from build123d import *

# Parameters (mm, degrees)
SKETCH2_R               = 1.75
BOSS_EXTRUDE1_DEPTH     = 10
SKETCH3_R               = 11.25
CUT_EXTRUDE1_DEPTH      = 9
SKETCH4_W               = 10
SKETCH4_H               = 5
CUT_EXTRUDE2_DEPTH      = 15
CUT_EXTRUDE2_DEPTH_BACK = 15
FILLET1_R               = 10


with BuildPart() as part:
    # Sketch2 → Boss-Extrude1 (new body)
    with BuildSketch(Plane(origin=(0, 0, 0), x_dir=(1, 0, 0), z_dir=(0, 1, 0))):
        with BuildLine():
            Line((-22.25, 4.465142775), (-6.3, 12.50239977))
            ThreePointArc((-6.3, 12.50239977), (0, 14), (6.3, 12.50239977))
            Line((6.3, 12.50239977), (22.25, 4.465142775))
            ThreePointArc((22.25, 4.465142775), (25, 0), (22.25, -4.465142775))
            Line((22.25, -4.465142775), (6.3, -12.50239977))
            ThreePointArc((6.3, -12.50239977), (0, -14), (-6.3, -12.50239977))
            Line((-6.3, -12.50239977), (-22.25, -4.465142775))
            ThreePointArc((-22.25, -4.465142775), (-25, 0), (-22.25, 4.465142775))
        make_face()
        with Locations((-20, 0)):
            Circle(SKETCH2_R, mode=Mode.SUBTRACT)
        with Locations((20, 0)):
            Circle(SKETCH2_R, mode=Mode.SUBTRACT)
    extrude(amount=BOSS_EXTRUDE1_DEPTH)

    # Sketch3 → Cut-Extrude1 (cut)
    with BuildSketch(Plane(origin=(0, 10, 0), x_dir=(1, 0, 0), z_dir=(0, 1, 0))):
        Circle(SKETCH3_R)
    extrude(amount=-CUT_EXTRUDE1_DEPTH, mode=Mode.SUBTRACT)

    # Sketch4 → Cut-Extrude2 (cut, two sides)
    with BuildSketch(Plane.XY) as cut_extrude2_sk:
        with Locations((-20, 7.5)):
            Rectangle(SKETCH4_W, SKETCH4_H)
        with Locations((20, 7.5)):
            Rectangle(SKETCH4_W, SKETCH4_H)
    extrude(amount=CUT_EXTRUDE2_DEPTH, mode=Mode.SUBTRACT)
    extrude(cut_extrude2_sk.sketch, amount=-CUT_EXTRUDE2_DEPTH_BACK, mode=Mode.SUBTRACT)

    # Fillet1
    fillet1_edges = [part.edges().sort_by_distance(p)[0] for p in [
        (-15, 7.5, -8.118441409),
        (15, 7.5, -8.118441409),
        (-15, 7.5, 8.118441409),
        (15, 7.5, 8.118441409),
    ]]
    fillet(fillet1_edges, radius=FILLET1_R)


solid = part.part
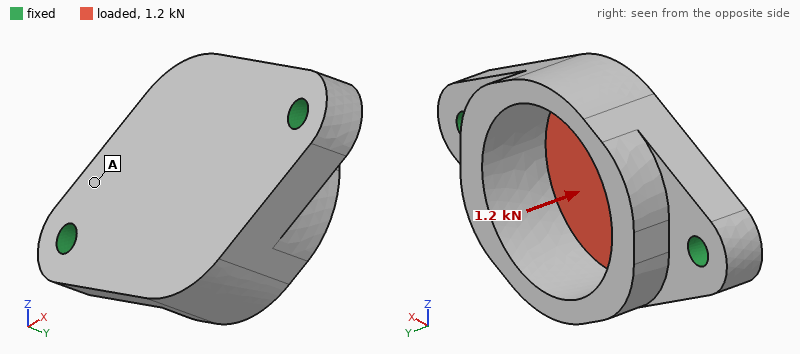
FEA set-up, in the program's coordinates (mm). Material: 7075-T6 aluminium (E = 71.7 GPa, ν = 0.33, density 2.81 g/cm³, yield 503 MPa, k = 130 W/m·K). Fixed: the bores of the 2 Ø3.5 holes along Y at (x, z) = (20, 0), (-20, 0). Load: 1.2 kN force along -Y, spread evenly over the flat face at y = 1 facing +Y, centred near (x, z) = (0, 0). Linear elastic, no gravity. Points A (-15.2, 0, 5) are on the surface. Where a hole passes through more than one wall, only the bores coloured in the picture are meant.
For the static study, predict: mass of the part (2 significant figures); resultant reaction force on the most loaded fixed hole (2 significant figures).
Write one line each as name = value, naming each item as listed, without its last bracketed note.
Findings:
mass of the part = 12 g
resultant reaction force on the most loaded fixed hole = 610 N
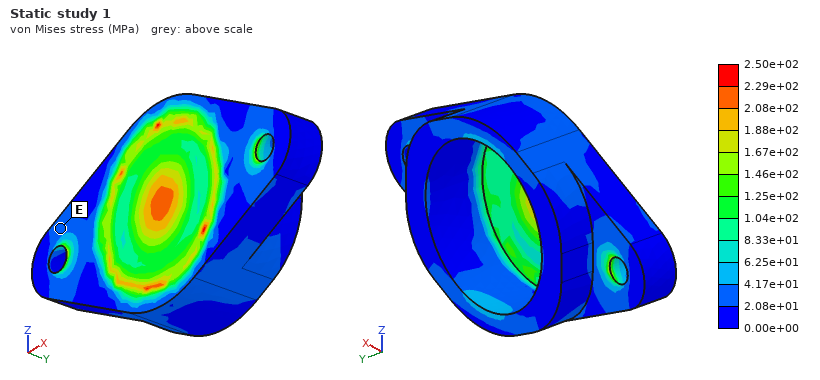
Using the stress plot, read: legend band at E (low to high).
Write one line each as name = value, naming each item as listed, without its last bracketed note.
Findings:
legend band at E = 2.08e+01 to 4.17e+01 MPa
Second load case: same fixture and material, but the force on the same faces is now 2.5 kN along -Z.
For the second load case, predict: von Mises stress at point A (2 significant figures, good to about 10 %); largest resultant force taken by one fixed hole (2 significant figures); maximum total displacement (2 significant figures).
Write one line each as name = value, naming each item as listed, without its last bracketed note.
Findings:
von Mises stress at point A = 42 MPa
largest resultant force taken by one fixed hole = 1.3 kN
maximum total displacement = 28 µm
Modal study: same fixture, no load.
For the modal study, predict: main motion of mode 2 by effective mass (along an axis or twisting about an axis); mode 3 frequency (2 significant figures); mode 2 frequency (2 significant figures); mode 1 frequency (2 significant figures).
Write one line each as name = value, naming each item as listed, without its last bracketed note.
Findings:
main motion of mode 2 by effective mass = along Y
mode 3 frequency = 19 kHz
mode 2 frequency = 13 kHz
mode 1 frequency = 11 kHz
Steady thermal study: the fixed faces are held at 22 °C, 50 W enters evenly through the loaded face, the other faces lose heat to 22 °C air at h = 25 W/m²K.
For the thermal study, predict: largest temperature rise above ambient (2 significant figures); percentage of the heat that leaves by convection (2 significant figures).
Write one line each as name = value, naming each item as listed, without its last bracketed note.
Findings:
largest temperature rise above ambient = 63 K
percentage of the heat that leaves by convection = 3.7 %
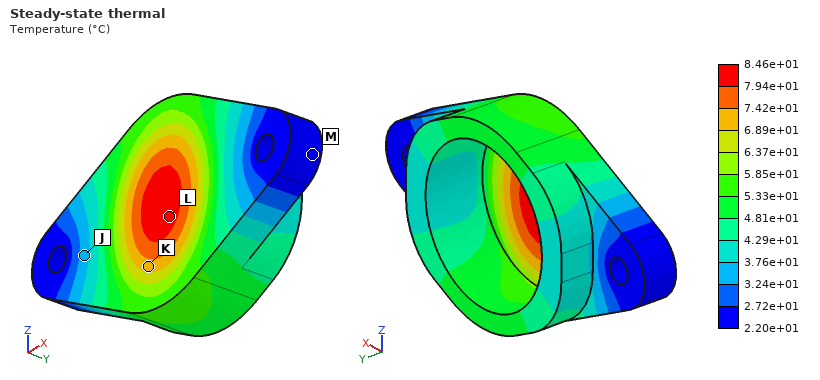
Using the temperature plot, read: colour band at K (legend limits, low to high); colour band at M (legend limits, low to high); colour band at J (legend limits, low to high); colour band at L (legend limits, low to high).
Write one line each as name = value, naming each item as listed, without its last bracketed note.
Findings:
colour band at K = 6.89e+01 to 7.42e+01 °C
colour band at M = 2.20e+01 to 2.72e+01 °C
colour band at J = 3.24e+01 to 3.76e+01 °C
colour band at L = 7.94e+01 to 8.46e+01 °C
